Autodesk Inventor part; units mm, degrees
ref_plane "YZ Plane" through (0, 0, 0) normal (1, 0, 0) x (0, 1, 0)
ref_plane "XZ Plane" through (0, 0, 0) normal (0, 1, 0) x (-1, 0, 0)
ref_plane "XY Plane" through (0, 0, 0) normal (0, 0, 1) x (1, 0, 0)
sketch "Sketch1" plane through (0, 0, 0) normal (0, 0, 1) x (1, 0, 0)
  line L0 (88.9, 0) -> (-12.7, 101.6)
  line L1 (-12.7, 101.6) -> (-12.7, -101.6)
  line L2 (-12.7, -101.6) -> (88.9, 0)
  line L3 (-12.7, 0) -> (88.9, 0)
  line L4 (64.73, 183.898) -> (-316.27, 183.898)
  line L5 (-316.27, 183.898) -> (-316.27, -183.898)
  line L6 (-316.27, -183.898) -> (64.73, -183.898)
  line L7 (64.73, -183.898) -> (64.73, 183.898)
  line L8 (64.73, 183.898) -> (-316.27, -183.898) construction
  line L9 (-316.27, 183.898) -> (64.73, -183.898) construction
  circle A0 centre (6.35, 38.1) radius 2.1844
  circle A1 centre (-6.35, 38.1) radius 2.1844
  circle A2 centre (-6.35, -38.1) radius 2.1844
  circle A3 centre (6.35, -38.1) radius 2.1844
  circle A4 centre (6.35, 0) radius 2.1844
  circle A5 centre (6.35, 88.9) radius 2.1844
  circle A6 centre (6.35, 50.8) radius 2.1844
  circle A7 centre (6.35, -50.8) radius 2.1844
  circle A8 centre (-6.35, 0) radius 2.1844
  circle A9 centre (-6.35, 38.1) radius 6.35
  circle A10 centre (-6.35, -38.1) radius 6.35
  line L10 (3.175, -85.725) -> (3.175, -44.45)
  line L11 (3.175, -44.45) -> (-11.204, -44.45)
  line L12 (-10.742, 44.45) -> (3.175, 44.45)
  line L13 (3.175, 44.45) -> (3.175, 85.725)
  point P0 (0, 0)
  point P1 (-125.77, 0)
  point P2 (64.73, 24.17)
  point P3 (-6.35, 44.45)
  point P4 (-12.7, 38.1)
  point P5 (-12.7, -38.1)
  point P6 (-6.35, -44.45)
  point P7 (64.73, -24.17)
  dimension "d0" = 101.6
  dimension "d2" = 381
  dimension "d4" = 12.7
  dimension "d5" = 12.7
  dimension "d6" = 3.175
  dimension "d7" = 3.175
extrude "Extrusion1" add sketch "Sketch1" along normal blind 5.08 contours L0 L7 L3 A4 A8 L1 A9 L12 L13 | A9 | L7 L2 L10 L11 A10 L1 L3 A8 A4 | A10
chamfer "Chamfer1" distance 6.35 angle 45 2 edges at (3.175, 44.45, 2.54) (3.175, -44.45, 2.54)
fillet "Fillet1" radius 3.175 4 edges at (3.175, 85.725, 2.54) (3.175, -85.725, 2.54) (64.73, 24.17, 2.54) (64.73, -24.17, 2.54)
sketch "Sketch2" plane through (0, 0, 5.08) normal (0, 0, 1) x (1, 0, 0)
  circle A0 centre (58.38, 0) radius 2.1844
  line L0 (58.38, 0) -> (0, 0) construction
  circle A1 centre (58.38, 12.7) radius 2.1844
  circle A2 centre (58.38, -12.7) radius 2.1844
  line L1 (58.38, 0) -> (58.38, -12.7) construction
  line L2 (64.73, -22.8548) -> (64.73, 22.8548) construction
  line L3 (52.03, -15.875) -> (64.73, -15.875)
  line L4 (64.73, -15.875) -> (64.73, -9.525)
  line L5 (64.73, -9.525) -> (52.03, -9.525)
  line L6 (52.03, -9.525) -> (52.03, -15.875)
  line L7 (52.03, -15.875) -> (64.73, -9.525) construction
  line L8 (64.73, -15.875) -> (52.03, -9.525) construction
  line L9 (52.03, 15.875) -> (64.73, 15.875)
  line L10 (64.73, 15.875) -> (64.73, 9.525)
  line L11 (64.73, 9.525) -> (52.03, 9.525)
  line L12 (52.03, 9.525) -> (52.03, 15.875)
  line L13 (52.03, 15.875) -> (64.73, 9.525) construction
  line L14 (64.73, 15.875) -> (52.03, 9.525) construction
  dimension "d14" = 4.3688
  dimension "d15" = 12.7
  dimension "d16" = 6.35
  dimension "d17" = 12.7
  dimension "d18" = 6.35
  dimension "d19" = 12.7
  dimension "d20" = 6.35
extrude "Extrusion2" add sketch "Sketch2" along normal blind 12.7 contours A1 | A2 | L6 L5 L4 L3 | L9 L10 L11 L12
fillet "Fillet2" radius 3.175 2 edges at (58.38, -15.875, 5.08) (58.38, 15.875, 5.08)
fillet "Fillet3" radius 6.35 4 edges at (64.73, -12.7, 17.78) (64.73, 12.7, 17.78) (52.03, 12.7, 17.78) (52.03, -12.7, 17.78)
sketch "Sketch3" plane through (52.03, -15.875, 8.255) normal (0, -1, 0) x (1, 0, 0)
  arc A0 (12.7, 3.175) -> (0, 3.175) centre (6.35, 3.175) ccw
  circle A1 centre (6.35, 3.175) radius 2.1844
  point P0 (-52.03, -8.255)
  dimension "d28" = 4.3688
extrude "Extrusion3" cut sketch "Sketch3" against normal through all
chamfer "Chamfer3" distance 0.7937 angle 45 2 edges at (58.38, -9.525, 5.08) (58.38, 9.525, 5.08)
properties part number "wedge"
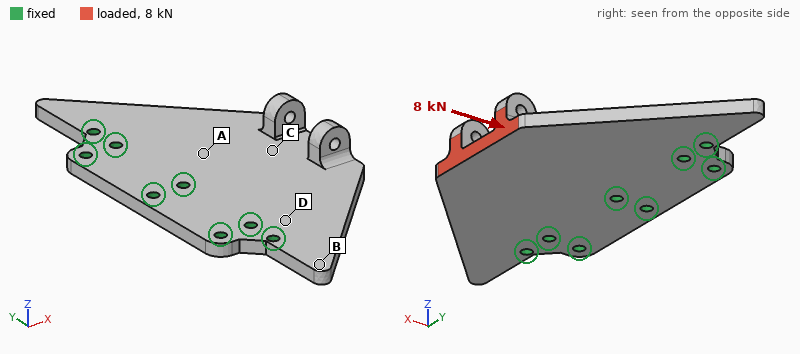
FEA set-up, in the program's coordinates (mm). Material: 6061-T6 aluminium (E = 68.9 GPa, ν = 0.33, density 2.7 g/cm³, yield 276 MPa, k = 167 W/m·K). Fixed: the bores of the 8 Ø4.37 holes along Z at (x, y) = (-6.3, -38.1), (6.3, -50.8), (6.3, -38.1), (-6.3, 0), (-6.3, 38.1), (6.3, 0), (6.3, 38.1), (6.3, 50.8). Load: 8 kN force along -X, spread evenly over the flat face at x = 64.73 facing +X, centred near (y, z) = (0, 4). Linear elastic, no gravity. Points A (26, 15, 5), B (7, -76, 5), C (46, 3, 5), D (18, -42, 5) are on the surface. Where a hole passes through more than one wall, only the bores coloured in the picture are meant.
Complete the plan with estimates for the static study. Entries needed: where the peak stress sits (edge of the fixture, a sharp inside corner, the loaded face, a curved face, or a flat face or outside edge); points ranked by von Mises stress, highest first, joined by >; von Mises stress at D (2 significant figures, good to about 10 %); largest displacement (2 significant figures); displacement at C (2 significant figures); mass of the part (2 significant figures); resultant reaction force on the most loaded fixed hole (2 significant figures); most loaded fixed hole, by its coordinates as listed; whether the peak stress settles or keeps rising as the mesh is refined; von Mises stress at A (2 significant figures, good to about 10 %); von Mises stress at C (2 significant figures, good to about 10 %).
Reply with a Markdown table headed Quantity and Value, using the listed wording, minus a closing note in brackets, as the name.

| Quantity | Value |
|---|---|
| where the peak stress sits | edge of the fixture |
| points ranked by von Mises stress, highest first, joined by > | C > A > D > B |
| von Mises stress at D | 33 MPa |
| largest displacement | 0.30 mm |
| displacement at C | 0.13 mm |
| mass of the part | 120 g |
| resultant reaction force on the most loaded fixed hole | 2.5 kN |
| most loaded fixed hole, by its coordinates as listed | (6.3, 0) |
| whether the peak stress settles or keeps rising as the mesh is refined | keeps rising |
| von Mises stress at A | 44 MPa |
| von Mises stress at C | 62 MPa |
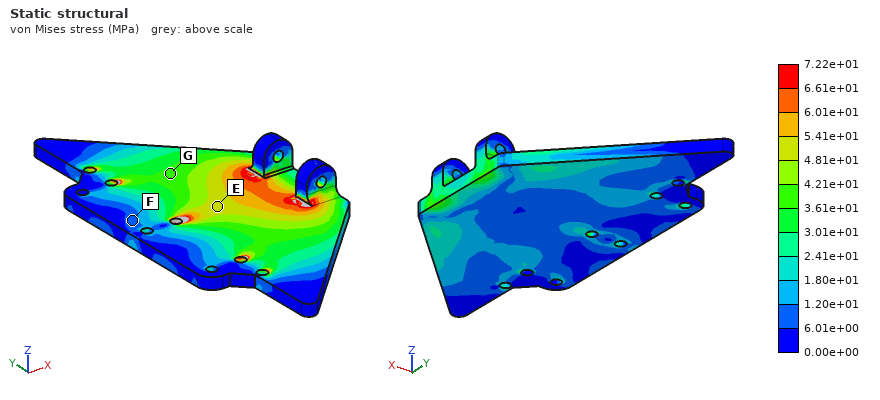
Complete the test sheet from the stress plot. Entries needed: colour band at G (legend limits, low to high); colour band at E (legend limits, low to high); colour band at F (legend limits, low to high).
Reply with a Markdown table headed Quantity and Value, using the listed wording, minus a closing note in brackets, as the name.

| Quantity | Value |
|---|---|
| colour band at G | 3.61e+01 to 4.21e+01 MPa |
| colour band at E | 4.81e+01 to 5.41e+01 MPa |
| colour band at F | 6.01e+00 to 1.20e+01 MPa |
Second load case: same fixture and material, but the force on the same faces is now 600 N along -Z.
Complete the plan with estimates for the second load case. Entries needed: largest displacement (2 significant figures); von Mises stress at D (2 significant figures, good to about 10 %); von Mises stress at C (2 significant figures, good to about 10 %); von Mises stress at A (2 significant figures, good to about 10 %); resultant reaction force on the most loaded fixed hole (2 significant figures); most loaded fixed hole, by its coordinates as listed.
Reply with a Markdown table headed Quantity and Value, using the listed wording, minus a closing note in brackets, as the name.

| Quantity | Value |
|---|---|
| largest displacement | 0.55 mm |
| von Mises stress at D | 47 MPa |
| von Mises stress at C | 34 MPa |
| von Mises stress at A | 49 MPa |
| resultant reaction force on the most loaded fixed hole | 770 N |
| most loaded fixed hole, by its coordinates as listed | (6.3, 0) |
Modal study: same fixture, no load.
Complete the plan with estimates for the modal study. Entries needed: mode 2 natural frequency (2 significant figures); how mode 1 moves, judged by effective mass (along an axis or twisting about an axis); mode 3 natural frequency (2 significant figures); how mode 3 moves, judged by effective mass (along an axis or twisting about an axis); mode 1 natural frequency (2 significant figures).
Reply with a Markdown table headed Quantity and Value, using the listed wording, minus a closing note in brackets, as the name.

| Quantity | Value |
|---|---|
| mode 2 natural frequency | 3000 Hz |
| how mode 1 moves, judged by effective mass | along Z |
| mode 3 natural frequency | 5400 Hz |
| how mode 3 moves, judged by effective mass | along Z |
| mode 1 natural frequency | 1300 Hz |
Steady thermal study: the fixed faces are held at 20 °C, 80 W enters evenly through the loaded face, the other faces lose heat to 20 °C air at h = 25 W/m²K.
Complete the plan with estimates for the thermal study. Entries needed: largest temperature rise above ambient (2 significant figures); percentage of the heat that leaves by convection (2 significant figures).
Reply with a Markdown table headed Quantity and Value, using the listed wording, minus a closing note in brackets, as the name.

| Quantity | Value |
|---|---|
| largest temperature rise above ambient | 68 K |
| percentage of the heat that leaves by convection | 11 % |
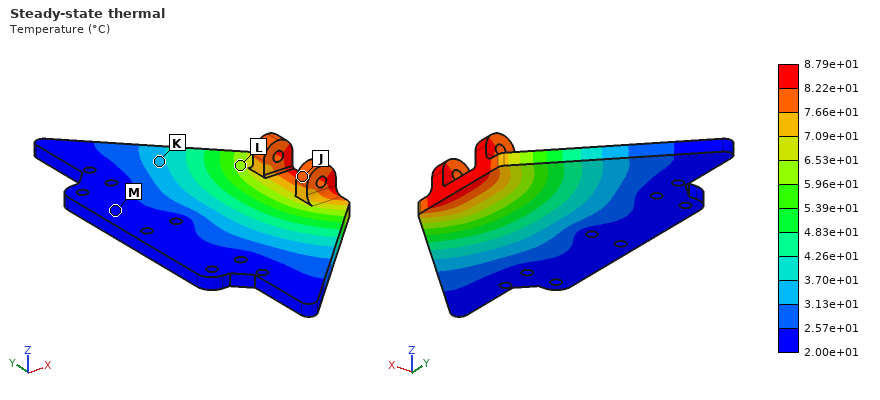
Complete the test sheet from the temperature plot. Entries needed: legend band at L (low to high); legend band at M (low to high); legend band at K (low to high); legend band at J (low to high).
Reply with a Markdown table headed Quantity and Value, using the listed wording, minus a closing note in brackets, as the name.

| Quantity | Value |
|---|---|
| legend band at L | 5.96e+01 to 6.53e+01 °C |
| legend band at M | 2.00e+01 to 2.57e+01 °C |
| legend band at K | 3.13e+01 to 3.70e+01 °C |
| legend band at J | 7.66e+01 to 8.22e+01 °C |
